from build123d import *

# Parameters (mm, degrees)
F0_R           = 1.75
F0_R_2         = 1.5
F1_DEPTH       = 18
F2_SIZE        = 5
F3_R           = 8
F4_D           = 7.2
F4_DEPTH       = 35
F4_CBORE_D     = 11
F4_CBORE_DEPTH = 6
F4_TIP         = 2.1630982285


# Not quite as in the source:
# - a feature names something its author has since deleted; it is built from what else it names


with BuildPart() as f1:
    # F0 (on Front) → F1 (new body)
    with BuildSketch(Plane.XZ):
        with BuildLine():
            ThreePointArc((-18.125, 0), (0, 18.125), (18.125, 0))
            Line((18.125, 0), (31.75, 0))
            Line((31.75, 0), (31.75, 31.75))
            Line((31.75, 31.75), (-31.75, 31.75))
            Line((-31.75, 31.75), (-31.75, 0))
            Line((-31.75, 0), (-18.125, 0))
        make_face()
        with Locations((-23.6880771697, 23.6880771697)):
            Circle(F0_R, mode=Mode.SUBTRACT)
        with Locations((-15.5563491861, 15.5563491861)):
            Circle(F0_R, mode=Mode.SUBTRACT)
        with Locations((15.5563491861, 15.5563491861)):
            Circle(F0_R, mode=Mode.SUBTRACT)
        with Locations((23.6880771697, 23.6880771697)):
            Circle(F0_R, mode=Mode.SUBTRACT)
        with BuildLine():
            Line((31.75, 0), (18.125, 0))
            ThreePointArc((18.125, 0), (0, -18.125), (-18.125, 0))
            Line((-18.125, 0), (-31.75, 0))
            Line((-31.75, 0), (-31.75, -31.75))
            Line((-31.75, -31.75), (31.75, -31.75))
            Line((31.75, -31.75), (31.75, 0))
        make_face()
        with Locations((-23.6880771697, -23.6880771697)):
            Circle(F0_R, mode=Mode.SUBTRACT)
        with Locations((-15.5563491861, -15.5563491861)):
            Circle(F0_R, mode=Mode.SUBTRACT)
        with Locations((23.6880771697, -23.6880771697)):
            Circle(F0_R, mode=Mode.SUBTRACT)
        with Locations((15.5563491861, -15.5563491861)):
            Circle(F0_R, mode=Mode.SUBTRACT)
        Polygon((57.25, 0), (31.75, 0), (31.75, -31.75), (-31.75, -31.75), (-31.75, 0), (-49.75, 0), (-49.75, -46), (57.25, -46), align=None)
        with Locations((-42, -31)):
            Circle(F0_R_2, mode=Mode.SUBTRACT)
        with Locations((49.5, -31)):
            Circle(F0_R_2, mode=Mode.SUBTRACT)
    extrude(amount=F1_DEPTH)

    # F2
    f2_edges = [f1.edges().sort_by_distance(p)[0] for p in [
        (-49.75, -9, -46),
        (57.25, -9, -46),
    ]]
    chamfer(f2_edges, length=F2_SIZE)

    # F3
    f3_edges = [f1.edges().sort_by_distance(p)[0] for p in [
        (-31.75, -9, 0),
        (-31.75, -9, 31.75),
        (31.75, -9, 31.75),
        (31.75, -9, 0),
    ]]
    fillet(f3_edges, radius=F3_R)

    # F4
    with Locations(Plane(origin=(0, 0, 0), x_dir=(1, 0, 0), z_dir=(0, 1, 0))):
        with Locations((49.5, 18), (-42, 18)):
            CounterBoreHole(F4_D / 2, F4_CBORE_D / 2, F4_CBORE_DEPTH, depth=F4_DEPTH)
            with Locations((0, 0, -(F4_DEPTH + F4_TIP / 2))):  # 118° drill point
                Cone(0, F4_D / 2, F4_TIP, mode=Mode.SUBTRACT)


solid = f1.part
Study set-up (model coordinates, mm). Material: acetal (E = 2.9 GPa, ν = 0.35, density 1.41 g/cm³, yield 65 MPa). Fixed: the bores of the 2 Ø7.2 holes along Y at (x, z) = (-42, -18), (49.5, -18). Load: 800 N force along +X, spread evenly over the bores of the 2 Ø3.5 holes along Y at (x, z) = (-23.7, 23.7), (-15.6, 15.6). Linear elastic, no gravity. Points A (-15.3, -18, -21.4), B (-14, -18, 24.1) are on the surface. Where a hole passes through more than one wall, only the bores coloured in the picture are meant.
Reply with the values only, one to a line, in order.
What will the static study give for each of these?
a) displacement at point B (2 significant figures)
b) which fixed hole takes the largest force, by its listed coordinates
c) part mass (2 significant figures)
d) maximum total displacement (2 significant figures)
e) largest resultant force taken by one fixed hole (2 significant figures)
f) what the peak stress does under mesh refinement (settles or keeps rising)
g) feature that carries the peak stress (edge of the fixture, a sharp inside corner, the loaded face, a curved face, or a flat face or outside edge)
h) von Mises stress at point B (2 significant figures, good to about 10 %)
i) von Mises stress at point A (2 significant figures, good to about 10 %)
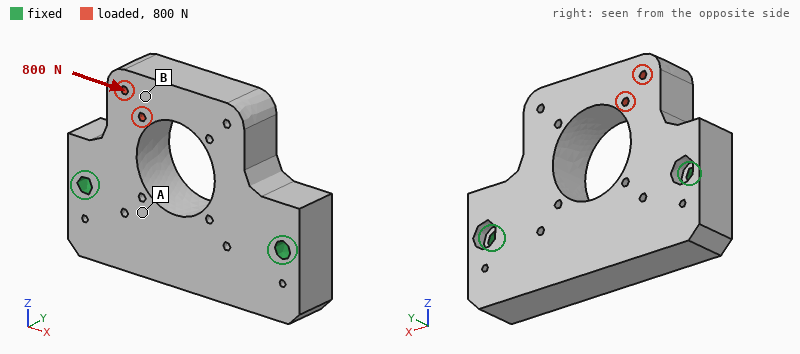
91 µm
(-42, -18)
140 g
98 µm
580 N
keeps rising
edge of the fixture
2.1 MPa
0.80 MPa
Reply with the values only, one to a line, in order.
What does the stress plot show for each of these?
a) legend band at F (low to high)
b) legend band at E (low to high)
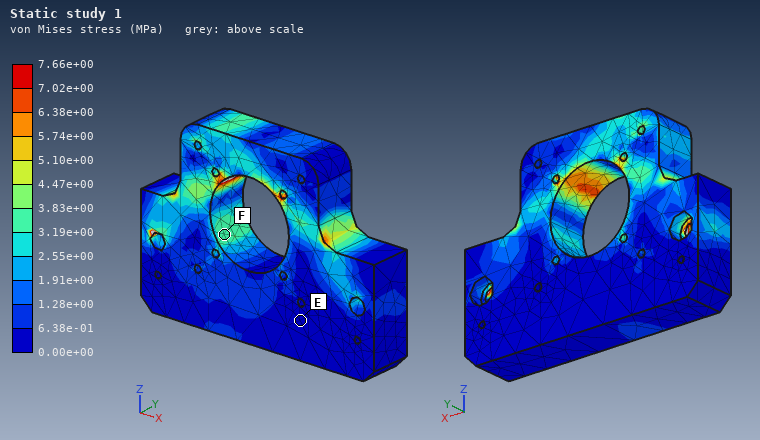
3.19e+00 to 3.83e+00 MPa
0.00e+00 to 6.38e-01 MPa
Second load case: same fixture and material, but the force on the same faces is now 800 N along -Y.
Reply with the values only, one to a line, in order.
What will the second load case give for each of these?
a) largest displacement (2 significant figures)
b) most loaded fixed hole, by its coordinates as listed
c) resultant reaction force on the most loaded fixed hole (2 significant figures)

0.96 mm
(-42, -18)
660 N
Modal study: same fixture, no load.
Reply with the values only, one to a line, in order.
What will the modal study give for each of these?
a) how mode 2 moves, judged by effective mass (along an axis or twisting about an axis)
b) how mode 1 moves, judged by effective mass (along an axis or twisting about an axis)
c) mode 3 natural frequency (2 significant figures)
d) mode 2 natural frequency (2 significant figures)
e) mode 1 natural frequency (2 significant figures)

along Y
along Y
2200 Hz
1700 Hz
910 Hz
